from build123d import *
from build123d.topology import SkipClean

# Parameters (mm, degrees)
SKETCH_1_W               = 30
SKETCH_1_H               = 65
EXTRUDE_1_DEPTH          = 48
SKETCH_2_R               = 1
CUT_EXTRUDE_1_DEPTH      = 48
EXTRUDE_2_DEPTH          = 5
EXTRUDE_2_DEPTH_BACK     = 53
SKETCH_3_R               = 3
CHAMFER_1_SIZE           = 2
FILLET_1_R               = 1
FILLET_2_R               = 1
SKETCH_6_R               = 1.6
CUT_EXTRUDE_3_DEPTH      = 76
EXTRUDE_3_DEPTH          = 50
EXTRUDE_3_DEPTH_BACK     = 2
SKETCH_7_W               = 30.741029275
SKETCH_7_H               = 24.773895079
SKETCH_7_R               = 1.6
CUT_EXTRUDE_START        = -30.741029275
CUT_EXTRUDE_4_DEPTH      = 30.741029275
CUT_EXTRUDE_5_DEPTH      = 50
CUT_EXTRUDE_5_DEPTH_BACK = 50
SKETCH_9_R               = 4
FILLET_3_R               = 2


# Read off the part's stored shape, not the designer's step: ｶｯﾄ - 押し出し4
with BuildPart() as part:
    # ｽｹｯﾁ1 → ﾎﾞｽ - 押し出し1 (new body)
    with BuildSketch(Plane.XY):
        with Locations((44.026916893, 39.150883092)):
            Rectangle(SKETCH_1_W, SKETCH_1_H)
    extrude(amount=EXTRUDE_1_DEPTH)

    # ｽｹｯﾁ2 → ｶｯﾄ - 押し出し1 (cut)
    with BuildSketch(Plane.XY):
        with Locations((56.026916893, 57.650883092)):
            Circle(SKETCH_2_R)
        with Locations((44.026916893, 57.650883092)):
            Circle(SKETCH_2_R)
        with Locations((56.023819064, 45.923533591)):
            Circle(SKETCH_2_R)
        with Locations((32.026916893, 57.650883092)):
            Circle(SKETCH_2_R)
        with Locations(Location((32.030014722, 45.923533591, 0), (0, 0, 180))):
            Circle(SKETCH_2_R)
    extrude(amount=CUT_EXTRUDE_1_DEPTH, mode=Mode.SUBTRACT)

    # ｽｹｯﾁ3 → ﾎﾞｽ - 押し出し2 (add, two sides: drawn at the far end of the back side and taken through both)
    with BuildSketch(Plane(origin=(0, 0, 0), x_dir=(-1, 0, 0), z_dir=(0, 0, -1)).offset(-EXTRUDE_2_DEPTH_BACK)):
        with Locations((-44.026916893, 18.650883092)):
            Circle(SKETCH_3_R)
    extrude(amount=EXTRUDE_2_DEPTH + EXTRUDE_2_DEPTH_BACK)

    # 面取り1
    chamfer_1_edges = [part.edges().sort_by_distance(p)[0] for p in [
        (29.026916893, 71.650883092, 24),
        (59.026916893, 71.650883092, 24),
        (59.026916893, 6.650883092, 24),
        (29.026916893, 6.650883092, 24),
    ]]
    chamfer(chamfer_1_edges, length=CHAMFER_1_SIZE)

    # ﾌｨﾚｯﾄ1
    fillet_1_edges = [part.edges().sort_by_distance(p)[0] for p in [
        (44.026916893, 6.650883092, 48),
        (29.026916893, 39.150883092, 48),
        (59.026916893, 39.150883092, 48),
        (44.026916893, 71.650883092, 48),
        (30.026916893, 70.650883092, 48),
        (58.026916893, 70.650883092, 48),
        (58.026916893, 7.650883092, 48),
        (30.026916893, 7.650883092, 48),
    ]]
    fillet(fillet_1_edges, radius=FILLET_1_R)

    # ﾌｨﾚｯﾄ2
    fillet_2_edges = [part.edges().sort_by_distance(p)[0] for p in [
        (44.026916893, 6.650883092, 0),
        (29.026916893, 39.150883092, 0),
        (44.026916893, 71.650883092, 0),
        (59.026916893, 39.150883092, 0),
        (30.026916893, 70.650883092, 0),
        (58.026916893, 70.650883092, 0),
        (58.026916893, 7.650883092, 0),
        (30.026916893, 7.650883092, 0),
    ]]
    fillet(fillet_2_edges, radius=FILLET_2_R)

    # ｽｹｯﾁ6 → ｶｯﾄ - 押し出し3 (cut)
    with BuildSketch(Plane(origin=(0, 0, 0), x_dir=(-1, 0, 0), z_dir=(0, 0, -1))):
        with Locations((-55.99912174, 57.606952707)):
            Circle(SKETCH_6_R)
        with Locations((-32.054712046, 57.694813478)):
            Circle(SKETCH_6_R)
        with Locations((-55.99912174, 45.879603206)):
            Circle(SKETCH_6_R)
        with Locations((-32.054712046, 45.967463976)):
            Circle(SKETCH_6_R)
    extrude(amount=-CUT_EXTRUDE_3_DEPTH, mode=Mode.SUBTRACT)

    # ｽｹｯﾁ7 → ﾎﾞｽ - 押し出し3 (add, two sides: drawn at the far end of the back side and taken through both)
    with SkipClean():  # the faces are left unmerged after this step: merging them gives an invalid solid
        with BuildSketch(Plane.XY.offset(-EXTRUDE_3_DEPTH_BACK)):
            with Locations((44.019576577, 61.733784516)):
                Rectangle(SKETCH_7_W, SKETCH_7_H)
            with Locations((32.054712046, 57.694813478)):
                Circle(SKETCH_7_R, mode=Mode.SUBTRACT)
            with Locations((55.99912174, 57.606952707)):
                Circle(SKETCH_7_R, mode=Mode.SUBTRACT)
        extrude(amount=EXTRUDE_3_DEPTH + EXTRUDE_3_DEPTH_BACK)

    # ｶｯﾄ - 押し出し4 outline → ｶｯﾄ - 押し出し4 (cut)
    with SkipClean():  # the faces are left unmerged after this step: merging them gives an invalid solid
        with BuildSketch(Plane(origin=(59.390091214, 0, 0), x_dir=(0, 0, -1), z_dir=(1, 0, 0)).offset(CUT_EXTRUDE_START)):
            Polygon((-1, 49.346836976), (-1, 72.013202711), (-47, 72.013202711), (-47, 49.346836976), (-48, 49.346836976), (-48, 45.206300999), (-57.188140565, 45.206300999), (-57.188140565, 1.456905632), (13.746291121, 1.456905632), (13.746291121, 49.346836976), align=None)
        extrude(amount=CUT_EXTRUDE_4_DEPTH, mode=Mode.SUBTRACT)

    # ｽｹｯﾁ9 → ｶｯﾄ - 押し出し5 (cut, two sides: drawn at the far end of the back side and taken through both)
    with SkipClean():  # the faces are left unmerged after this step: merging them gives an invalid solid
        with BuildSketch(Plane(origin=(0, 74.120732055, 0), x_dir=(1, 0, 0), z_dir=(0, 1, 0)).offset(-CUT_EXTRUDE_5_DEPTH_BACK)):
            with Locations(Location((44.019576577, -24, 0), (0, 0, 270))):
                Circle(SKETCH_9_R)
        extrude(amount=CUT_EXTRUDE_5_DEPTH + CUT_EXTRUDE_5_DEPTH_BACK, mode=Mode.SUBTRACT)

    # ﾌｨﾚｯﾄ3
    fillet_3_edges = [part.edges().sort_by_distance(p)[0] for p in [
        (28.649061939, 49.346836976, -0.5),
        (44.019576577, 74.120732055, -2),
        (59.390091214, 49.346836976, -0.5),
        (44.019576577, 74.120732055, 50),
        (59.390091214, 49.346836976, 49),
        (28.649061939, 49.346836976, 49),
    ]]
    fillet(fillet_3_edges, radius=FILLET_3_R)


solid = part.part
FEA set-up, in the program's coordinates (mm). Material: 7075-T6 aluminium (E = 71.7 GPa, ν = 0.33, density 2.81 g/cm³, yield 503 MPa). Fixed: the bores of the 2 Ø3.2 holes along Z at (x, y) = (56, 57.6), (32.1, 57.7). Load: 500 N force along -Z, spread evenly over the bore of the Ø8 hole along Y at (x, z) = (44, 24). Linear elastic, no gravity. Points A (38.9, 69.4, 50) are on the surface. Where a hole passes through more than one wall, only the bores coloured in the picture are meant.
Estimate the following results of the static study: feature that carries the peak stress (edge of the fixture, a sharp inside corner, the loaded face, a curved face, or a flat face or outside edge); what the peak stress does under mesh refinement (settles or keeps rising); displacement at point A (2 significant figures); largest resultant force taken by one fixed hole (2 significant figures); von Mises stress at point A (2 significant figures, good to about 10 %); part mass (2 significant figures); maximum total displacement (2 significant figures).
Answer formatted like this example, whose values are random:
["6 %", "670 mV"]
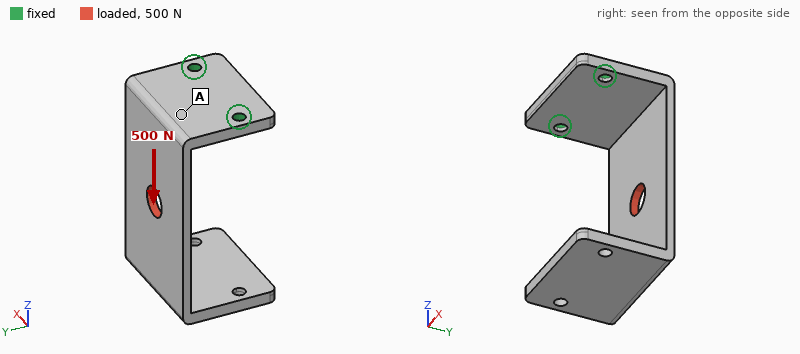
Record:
["edge of the fixture", "keeps rising", "0.12 mm", "260 N", "41 MPa", "20 g", "0.75 mm"]
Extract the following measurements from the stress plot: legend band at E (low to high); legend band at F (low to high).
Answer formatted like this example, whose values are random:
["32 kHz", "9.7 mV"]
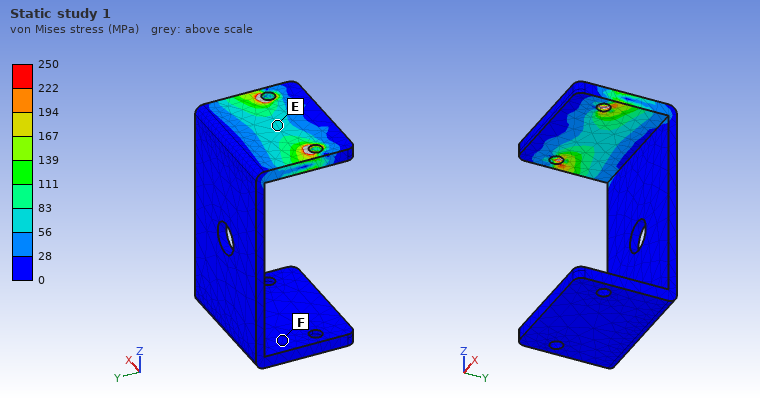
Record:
["56 to 83 MPa", "0 to 28 MPa"]
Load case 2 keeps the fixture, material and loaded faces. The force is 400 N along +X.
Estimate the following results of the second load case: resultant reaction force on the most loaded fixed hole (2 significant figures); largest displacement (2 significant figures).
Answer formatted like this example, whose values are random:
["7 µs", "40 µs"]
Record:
["520 N", "0.70 mm"]
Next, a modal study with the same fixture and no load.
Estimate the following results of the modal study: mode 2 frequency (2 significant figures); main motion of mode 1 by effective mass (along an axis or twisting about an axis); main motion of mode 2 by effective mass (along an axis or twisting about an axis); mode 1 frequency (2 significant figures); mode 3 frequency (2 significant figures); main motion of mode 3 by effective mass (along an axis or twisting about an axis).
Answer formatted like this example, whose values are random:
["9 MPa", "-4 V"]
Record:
["730 Hz", "along Y", "along X", "310 Hz", "1300 Hz", "along Z"]
